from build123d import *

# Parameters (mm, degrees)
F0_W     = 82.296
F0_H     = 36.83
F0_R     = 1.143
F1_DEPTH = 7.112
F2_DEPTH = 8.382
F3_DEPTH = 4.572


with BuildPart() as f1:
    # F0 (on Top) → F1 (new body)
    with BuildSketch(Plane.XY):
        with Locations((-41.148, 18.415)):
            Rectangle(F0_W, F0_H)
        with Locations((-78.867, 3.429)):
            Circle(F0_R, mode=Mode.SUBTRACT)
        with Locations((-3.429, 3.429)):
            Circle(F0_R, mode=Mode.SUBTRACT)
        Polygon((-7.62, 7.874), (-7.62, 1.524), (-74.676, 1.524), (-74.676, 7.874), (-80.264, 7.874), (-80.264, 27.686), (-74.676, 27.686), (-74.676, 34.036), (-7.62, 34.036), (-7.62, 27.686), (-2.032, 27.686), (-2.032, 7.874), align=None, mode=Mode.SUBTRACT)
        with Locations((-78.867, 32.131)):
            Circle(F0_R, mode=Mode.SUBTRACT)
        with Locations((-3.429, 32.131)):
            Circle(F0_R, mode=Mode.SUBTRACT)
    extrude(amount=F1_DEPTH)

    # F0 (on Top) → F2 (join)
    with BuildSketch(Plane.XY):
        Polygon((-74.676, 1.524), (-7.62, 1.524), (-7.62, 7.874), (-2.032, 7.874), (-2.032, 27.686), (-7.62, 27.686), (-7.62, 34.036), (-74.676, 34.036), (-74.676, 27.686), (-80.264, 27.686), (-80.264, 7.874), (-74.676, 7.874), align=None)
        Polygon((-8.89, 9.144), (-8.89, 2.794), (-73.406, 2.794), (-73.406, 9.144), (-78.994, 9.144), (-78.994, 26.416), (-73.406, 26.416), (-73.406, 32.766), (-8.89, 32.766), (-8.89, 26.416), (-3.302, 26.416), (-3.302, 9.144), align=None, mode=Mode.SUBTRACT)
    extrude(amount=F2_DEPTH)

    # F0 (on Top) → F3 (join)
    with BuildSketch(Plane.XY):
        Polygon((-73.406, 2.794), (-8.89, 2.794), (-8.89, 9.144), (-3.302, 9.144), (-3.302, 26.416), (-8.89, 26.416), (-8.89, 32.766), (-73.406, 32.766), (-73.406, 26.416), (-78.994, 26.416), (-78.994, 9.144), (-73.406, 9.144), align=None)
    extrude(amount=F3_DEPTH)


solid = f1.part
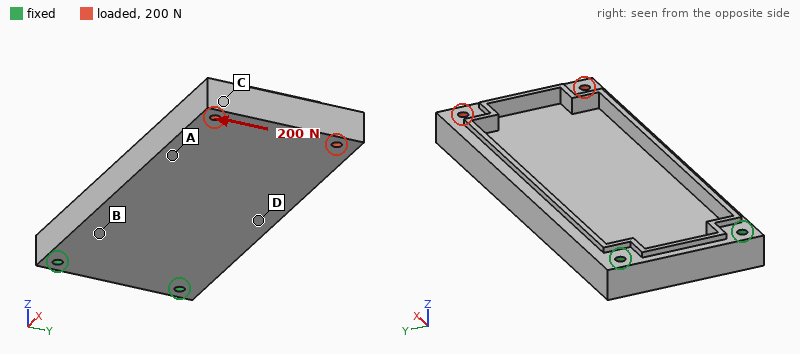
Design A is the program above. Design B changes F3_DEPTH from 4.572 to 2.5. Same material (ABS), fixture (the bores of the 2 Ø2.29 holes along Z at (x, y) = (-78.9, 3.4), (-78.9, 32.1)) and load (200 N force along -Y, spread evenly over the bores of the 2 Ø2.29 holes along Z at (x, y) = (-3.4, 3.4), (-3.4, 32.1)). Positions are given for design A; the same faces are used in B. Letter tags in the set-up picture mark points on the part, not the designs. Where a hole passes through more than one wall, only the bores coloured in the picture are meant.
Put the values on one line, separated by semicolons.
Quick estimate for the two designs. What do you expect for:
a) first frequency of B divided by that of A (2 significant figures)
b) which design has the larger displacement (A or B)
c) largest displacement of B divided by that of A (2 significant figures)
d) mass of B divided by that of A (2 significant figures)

1.0; B; 2.8; 0.73
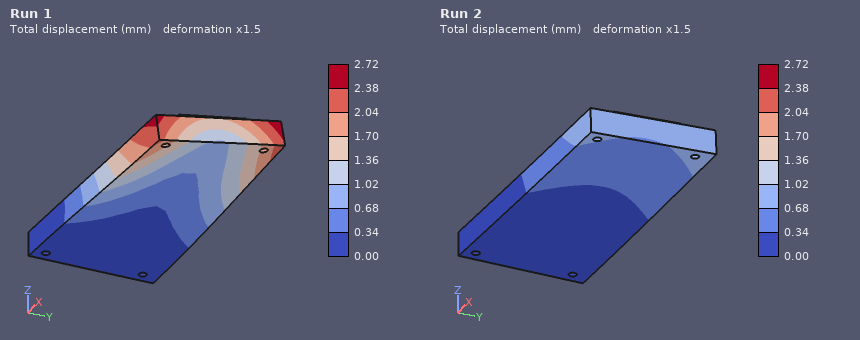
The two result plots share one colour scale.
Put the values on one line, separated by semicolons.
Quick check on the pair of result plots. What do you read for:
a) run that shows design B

Run 1
